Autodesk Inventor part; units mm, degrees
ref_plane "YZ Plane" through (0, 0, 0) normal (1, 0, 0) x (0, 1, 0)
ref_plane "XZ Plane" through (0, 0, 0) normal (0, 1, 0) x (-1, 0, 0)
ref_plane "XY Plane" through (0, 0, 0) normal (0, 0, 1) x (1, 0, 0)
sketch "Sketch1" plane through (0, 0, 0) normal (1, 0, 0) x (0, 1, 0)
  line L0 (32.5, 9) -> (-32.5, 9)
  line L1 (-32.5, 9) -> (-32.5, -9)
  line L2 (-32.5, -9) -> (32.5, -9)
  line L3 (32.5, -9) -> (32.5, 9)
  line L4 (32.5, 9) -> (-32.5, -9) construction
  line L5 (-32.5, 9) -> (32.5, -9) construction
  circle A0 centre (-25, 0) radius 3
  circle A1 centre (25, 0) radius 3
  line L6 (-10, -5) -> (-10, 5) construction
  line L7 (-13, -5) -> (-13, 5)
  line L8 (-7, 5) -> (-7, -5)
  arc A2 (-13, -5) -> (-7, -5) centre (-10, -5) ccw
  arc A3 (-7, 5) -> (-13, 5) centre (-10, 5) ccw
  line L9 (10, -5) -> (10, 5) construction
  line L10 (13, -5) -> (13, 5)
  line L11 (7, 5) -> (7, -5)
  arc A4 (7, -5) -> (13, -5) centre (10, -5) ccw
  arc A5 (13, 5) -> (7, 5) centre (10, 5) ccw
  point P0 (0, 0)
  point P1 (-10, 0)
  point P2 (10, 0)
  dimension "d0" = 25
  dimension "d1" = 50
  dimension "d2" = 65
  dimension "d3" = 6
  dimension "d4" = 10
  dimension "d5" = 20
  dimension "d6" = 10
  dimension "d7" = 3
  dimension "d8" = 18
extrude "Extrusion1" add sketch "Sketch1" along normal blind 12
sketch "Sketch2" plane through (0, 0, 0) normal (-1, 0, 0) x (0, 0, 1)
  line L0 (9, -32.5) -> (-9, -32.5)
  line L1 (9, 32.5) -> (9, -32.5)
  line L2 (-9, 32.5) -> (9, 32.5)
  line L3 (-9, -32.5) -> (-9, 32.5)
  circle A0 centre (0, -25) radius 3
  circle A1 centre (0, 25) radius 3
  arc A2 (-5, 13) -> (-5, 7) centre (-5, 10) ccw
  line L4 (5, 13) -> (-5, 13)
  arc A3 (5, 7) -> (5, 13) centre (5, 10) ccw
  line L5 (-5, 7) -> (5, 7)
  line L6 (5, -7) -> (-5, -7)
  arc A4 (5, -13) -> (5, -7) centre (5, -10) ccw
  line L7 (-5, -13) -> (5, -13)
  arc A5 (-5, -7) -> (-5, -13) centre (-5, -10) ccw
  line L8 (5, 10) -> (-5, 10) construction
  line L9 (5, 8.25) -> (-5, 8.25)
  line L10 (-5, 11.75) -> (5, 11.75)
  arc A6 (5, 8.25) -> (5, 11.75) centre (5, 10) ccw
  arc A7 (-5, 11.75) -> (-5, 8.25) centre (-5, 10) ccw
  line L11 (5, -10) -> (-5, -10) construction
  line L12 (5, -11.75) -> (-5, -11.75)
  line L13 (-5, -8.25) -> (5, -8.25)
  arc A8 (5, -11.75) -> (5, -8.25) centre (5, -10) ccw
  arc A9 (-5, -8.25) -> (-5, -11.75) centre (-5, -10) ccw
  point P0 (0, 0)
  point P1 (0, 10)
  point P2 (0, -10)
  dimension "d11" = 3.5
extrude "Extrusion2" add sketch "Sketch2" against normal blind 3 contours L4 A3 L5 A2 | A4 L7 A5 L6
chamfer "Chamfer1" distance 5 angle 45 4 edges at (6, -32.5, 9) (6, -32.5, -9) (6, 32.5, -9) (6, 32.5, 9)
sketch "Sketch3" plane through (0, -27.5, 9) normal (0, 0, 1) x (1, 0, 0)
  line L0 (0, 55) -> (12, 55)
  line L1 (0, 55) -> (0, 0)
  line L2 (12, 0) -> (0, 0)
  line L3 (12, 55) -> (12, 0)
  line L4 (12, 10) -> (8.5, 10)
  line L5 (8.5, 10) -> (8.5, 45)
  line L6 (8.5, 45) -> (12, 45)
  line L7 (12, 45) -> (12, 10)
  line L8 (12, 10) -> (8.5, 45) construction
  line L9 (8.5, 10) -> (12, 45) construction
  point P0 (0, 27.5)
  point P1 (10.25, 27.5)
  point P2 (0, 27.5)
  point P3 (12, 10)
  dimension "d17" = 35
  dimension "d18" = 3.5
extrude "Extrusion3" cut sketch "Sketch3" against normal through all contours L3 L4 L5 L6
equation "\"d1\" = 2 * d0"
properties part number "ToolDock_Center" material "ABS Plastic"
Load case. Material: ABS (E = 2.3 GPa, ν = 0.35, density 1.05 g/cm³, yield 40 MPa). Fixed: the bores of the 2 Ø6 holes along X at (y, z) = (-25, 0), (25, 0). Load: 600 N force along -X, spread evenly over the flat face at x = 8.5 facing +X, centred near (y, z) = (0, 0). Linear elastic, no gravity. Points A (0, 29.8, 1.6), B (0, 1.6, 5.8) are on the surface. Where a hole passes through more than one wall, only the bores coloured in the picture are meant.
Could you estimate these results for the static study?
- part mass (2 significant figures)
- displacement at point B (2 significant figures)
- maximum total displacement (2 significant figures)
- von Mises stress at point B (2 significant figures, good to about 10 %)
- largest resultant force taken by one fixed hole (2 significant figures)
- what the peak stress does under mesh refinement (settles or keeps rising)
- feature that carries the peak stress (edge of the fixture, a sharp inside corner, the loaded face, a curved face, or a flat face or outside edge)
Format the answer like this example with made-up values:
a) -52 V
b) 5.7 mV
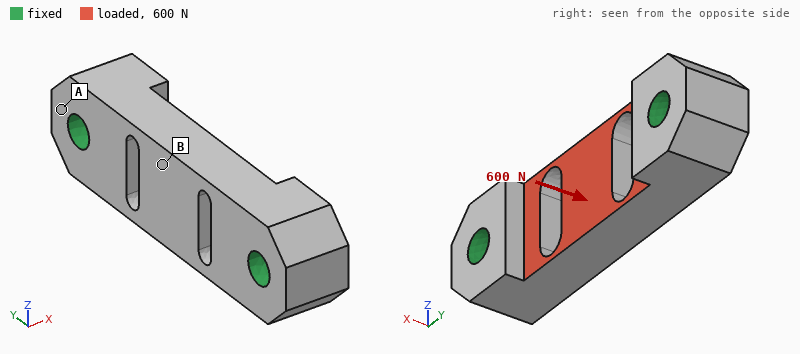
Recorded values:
a) 9.8 g
b) 0.20 mm
c) 0.21 mm
d) 7.3 MPa
e) 300 N
f) keeps rising
g) a sharp inside corner
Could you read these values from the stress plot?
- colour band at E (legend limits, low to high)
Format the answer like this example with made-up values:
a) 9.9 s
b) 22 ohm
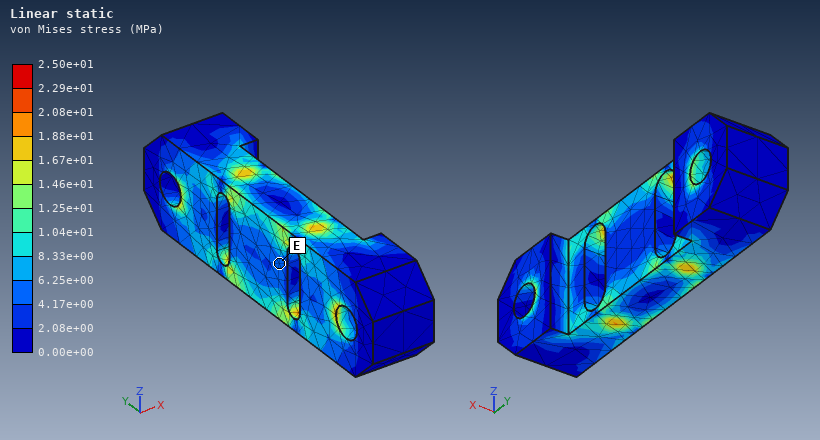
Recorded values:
a) 4.17e+00 to 6.25e+00 MPa
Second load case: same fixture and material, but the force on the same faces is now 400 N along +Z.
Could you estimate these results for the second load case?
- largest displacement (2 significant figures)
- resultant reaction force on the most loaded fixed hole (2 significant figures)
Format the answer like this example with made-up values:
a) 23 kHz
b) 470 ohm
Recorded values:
a) 0.25 mm
b) 200 N
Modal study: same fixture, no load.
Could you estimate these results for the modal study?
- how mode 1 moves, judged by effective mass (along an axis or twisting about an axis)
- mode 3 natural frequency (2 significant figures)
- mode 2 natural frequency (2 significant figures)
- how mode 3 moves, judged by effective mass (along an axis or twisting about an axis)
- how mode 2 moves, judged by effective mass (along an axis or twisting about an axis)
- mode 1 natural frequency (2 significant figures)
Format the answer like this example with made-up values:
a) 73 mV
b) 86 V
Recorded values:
a) along Z
b) 6700 Hz
c) 4400 Hz
d) twisting about Y
e) along X
f) 3900 Hz
